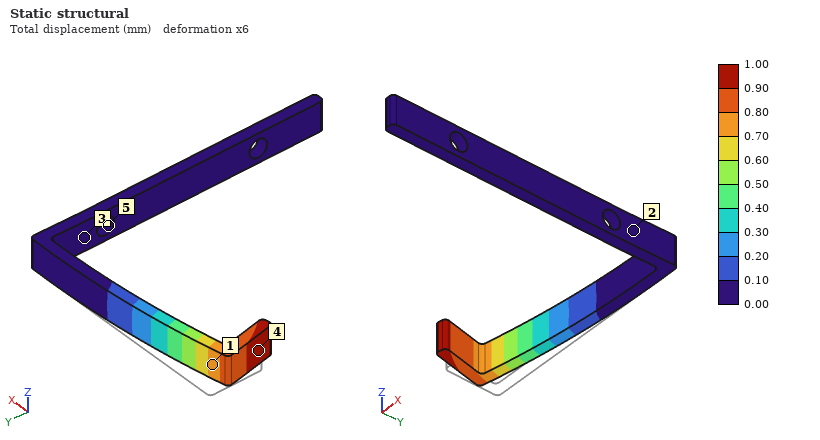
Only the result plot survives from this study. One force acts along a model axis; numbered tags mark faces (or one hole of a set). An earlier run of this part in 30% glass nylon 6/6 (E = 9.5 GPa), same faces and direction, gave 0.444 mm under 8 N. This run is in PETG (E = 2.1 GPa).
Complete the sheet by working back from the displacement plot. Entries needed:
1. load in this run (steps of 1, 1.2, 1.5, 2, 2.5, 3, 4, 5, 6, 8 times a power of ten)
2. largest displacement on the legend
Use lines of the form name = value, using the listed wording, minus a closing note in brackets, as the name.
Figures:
load in this run = 4 N
largest displacement on the legend = 1.00 mm
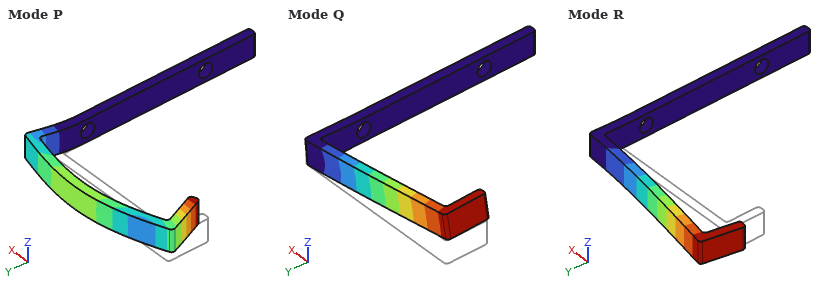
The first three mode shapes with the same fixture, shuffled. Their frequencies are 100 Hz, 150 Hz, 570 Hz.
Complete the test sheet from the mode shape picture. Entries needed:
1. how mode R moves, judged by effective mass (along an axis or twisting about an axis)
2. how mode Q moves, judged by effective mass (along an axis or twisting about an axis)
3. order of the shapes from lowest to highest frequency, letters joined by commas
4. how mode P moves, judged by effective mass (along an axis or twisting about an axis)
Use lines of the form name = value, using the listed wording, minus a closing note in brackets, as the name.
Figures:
how mode R moves, judged by effective mass = along Y
how mode Q moves, judged by effective mass = along Z
order of the shapes from lowest to highest frequency, letters joined by commas = R, Q, P
how mode P moves, judged by effective mass = along X
